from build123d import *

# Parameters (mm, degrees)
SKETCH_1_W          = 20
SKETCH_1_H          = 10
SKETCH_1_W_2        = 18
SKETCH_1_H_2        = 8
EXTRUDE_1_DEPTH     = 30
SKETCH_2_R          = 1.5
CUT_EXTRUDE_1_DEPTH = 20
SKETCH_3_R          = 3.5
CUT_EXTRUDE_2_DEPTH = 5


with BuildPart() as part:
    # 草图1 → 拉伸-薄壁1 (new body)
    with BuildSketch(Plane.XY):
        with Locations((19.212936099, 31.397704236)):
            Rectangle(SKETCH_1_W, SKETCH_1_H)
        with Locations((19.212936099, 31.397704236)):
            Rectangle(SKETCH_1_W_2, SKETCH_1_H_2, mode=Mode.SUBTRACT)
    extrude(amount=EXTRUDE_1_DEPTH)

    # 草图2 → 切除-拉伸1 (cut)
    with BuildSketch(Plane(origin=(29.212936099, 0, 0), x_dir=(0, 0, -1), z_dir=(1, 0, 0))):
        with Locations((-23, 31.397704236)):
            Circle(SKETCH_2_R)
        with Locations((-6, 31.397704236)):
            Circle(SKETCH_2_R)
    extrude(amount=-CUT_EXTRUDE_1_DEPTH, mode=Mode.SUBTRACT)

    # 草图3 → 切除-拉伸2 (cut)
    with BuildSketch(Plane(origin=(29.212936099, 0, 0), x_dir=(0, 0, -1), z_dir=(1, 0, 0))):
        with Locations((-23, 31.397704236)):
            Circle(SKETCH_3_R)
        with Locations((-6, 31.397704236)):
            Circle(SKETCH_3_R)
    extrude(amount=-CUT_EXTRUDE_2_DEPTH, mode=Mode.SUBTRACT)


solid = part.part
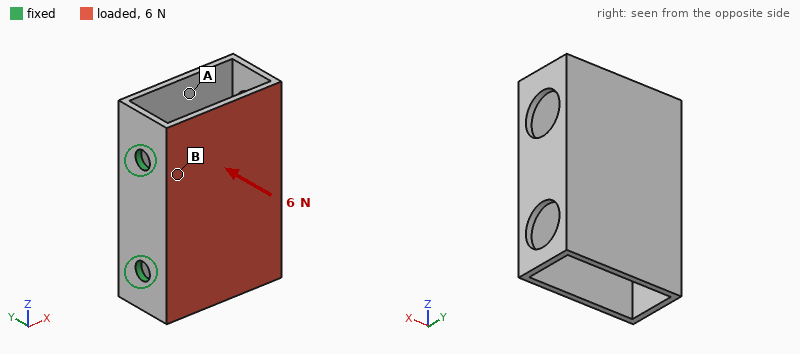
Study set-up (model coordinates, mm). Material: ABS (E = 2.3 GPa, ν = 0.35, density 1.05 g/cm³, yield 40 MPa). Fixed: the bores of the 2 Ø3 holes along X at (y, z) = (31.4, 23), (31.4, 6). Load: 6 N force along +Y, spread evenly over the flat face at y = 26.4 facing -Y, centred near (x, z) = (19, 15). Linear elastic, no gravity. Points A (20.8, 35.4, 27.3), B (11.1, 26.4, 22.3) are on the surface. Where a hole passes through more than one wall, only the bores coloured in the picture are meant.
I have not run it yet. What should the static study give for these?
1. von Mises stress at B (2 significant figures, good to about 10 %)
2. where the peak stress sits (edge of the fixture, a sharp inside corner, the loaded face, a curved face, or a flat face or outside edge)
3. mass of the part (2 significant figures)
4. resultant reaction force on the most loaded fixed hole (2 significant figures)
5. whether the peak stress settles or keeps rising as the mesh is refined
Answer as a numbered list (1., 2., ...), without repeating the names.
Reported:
1. 2.6 MPa
2. edge of the fixture
3. 1.7 g
4. 3.1 N
5. keeps rising
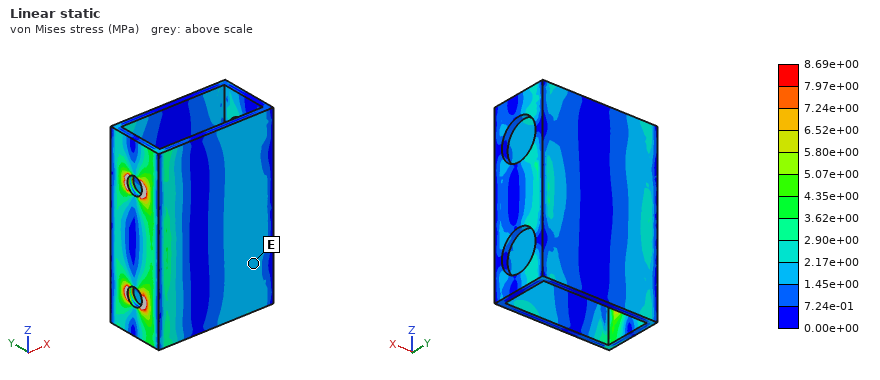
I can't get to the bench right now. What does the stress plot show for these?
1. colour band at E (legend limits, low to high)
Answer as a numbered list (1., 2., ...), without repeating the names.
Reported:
1. 1.45e+00 to 2.17e+00 MPa
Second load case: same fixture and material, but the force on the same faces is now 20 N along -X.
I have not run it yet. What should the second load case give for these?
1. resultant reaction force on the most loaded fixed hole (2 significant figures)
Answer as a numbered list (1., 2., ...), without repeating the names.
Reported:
1. 11 N
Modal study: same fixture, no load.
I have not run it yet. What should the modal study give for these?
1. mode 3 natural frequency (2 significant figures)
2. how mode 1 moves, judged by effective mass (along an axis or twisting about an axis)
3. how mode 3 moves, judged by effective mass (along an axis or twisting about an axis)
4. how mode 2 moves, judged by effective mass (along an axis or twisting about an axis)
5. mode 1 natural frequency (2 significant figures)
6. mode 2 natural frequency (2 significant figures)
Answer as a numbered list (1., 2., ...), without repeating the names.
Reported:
1. 2000 Hz
2. along Y
3. along Z
4. twisting about X
5. 560 Hz
6. 1800 Hz
